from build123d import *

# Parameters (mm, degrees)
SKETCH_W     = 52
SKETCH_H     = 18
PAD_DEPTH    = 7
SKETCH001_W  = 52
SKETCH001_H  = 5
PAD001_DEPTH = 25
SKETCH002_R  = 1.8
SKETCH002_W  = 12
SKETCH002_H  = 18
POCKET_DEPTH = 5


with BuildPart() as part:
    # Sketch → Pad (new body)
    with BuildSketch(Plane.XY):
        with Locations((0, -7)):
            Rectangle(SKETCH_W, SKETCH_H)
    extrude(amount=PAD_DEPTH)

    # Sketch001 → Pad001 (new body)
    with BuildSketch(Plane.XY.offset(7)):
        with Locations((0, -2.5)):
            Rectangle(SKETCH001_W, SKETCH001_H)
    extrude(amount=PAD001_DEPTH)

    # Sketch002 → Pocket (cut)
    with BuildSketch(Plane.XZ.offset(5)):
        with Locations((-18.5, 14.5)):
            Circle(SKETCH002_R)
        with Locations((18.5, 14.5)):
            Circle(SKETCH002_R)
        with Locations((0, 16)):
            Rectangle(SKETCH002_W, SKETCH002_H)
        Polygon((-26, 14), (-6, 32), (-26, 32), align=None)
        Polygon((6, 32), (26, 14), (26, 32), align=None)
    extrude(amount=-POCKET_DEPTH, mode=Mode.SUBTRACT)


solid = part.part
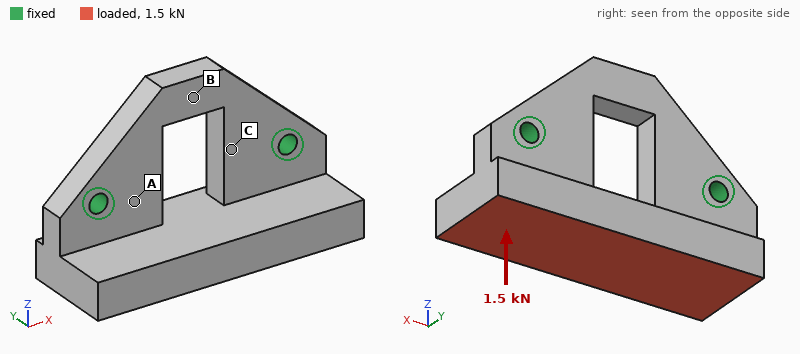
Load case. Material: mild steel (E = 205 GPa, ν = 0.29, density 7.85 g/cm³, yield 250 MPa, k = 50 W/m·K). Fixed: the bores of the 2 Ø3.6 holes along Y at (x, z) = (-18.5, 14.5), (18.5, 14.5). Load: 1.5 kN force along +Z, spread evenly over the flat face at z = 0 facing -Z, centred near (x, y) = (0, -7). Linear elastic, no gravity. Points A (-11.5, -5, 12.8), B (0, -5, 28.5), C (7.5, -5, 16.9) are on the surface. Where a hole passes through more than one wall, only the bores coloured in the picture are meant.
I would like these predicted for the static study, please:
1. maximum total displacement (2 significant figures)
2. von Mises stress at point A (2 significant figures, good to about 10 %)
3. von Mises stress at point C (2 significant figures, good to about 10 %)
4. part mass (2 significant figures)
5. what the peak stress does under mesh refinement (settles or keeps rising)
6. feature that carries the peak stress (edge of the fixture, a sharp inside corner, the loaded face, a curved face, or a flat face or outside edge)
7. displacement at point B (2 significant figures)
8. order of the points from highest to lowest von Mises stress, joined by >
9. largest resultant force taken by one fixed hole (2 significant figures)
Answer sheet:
16 µm
31 MPa
15 MPa
79 g
keeps rising
edge of the fixture
3.5 µm
A > C > B
760 N
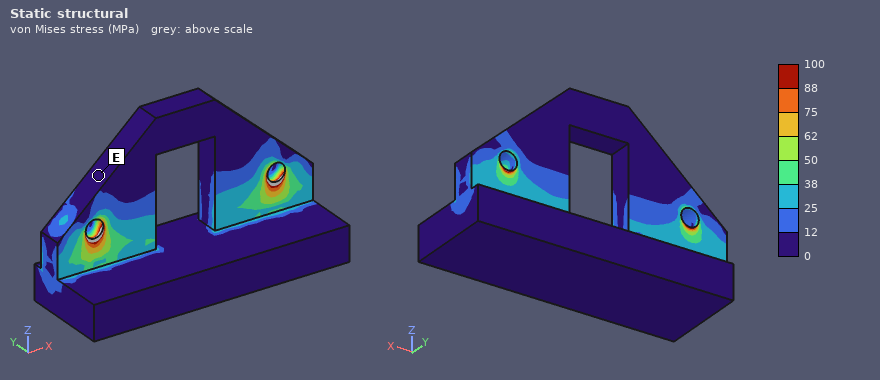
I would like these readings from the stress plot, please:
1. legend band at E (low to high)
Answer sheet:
0 to 12 MPa
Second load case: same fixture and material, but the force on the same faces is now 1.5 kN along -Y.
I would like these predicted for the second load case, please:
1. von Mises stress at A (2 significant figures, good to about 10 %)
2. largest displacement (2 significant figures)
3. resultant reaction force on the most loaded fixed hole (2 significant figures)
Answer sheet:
62 MPa
35 µm
750 N
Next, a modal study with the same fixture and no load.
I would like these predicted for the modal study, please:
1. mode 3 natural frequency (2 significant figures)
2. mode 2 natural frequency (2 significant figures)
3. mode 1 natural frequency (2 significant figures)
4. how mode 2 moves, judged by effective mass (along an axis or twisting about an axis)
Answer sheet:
12 kHz
11 kHz
6000 Hz
along Y
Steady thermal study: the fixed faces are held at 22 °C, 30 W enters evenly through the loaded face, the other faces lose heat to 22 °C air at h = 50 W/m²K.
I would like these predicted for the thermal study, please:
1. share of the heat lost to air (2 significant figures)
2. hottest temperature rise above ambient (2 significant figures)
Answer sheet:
13 %
41 K
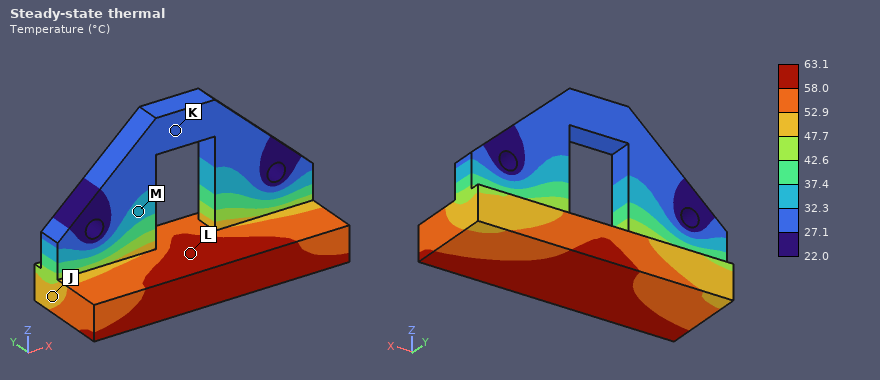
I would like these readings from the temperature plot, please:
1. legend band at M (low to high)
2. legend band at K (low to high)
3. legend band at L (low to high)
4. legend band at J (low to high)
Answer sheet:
32.3 to 37.4 °C
27.1 to 32.3 °C
58.0 to 63.1 °C
47.7 to 52.9 °C
